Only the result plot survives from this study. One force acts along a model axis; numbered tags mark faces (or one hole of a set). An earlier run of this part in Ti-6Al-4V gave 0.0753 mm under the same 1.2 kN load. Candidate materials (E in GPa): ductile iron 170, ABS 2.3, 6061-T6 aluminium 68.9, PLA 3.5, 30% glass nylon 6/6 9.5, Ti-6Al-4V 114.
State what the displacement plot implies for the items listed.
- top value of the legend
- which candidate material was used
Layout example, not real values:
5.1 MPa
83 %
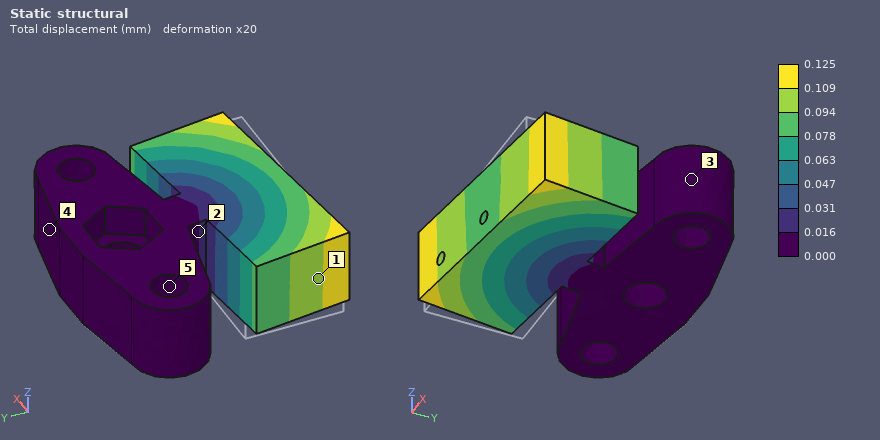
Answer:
0.125 mm
6061-T6 aluminium
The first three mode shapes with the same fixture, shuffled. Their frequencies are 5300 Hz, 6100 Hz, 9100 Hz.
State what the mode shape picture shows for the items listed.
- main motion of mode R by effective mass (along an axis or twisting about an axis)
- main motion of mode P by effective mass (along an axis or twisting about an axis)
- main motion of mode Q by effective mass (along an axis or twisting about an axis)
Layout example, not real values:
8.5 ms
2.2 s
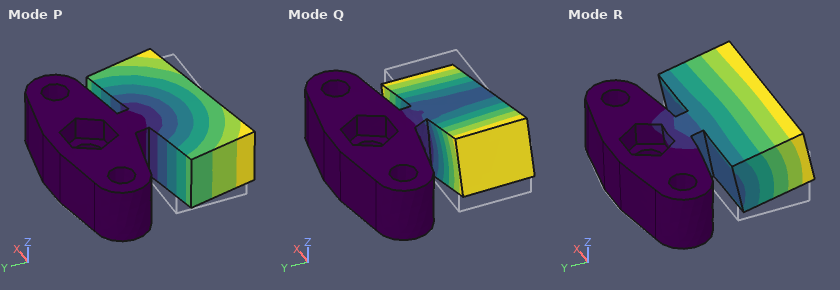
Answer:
along Z
along X
twisting about Y
